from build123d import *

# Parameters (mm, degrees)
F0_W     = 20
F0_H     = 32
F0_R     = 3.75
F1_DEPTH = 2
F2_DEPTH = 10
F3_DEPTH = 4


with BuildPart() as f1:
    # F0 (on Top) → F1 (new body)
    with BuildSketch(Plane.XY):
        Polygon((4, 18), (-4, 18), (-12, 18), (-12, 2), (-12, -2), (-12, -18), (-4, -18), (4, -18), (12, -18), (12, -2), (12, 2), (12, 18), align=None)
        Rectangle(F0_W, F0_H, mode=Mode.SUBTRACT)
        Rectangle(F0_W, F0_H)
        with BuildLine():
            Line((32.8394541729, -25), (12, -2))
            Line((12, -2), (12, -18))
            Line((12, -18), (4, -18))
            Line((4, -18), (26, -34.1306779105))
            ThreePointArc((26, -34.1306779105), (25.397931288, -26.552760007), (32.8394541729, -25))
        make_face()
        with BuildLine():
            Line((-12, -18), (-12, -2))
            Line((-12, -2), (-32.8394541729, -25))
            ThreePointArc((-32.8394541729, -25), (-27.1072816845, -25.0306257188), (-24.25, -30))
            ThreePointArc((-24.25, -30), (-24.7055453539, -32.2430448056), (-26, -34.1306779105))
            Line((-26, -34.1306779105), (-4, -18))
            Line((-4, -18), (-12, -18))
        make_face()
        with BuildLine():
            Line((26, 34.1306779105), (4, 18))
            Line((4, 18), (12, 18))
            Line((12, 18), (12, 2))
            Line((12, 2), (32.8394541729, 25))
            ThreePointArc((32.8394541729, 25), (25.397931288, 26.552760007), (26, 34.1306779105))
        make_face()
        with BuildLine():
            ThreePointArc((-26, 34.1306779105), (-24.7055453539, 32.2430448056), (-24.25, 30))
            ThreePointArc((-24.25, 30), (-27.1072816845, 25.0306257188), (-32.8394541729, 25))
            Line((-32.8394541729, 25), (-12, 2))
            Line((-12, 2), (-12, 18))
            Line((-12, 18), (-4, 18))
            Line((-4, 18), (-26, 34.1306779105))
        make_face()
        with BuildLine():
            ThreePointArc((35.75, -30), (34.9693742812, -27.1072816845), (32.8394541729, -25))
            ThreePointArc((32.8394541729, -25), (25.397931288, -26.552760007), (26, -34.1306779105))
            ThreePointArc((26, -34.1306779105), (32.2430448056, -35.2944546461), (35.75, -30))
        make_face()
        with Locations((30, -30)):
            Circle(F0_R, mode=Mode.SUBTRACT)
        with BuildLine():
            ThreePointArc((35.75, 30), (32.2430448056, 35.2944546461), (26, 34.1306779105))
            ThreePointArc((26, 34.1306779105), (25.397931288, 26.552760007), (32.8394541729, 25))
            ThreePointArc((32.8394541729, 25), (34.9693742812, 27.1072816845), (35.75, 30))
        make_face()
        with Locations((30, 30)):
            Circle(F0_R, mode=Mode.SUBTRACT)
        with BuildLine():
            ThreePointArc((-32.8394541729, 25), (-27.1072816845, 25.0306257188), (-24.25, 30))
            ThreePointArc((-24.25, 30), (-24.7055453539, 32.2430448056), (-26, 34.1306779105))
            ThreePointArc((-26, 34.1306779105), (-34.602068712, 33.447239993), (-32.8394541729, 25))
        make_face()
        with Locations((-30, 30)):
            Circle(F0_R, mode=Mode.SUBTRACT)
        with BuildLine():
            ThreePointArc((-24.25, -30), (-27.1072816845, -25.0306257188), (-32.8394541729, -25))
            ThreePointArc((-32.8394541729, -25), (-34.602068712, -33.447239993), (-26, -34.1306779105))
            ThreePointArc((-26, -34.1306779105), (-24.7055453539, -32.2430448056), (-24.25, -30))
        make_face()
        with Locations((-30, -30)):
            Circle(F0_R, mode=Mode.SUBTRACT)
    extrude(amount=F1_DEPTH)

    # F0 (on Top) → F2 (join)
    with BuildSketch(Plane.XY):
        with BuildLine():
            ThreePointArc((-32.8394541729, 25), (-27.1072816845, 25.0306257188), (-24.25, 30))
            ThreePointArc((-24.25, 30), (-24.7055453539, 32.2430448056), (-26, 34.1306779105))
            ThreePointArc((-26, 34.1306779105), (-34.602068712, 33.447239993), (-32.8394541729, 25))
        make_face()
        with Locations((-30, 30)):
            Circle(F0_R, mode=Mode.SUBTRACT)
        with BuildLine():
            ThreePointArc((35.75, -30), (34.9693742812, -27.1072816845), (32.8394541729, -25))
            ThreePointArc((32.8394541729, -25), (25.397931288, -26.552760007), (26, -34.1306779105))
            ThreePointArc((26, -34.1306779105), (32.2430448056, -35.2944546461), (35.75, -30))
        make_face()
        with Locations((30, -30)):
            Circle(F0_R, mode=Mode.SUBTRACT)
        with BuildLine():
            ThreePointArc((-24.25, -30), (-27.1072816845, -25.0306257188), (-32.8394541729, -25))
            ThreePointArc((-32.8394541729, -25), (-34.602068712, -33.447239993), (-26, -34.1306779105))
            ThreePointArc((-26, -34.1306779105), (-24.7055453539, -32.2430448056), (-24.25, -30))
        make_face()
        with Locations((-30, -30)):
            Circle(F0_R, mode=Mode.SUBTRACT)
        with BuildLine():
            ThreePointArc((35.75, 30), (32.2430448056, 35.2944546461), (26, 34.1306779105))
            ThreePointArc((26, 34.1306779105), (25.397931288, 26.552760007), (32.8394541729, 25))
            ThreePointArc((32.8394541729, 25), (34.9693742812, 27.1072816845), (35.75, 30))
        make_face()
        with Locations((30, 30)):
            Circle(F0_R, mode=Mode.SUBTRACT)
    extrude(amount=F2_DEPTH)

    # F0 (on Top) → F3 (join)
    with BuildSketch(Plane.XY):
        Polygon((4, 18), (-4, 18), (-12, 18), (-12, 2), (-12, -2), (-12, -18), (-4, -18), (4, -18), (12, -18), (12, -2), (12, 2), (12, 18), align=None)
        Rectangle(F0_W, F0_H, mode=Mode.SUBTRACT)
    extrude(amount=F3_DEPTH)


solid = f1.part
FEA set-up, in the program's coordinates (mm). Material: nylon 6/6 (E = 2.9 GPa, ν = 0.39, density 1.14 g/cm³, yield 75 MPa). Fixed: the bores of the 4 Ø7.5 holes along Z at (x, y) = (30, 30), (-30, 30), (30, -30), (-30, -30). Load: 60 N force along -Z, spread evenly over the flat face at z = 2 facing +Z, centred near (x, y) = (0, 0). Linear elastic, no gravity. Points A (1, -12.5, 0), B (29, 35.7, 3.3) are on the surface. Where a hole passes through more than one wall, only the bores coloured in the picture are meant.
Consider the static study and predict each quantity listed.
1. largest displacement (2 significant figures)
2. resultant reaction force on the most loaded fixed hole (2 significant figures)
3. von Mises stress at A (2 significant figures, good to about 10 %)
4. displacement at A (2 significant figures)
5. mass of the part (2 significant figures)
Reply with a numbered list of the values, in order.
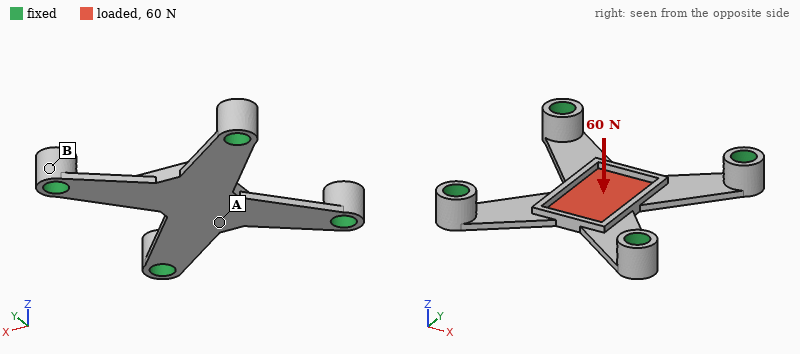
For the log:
1. 0.94 mm
2. 20 N
3. 7.8 MPa
4. 0.80 mm
5. 8.0 g
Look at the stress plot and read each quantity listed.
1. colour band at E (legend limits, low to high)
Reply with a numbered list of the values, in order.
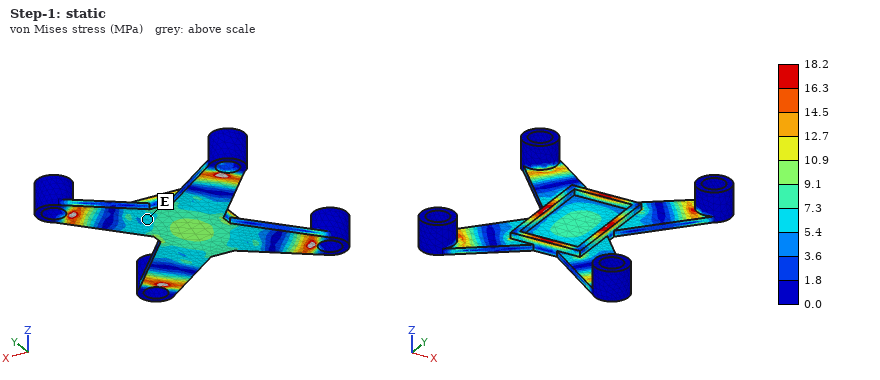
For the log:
1. 5.4 to 7.3 MPa
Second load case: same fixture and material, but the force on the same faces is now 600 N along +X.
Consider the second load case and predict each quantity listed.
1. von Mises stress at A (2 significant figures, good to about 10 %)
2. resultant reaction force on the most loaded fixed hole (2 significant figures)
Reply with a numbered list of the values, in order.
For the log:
1. 2.4 MPa
2. 190 N
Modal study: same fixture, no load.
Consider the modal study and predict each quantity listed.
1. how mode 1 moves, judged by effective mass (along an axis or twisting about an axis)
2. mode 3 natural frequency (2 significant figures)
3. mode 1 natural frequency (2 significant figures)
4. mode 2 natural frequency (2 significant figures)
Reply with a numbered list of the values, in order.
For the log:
1. along Z
2. 1700 Hz
3. 790 Hz
4. 1600 Hz
